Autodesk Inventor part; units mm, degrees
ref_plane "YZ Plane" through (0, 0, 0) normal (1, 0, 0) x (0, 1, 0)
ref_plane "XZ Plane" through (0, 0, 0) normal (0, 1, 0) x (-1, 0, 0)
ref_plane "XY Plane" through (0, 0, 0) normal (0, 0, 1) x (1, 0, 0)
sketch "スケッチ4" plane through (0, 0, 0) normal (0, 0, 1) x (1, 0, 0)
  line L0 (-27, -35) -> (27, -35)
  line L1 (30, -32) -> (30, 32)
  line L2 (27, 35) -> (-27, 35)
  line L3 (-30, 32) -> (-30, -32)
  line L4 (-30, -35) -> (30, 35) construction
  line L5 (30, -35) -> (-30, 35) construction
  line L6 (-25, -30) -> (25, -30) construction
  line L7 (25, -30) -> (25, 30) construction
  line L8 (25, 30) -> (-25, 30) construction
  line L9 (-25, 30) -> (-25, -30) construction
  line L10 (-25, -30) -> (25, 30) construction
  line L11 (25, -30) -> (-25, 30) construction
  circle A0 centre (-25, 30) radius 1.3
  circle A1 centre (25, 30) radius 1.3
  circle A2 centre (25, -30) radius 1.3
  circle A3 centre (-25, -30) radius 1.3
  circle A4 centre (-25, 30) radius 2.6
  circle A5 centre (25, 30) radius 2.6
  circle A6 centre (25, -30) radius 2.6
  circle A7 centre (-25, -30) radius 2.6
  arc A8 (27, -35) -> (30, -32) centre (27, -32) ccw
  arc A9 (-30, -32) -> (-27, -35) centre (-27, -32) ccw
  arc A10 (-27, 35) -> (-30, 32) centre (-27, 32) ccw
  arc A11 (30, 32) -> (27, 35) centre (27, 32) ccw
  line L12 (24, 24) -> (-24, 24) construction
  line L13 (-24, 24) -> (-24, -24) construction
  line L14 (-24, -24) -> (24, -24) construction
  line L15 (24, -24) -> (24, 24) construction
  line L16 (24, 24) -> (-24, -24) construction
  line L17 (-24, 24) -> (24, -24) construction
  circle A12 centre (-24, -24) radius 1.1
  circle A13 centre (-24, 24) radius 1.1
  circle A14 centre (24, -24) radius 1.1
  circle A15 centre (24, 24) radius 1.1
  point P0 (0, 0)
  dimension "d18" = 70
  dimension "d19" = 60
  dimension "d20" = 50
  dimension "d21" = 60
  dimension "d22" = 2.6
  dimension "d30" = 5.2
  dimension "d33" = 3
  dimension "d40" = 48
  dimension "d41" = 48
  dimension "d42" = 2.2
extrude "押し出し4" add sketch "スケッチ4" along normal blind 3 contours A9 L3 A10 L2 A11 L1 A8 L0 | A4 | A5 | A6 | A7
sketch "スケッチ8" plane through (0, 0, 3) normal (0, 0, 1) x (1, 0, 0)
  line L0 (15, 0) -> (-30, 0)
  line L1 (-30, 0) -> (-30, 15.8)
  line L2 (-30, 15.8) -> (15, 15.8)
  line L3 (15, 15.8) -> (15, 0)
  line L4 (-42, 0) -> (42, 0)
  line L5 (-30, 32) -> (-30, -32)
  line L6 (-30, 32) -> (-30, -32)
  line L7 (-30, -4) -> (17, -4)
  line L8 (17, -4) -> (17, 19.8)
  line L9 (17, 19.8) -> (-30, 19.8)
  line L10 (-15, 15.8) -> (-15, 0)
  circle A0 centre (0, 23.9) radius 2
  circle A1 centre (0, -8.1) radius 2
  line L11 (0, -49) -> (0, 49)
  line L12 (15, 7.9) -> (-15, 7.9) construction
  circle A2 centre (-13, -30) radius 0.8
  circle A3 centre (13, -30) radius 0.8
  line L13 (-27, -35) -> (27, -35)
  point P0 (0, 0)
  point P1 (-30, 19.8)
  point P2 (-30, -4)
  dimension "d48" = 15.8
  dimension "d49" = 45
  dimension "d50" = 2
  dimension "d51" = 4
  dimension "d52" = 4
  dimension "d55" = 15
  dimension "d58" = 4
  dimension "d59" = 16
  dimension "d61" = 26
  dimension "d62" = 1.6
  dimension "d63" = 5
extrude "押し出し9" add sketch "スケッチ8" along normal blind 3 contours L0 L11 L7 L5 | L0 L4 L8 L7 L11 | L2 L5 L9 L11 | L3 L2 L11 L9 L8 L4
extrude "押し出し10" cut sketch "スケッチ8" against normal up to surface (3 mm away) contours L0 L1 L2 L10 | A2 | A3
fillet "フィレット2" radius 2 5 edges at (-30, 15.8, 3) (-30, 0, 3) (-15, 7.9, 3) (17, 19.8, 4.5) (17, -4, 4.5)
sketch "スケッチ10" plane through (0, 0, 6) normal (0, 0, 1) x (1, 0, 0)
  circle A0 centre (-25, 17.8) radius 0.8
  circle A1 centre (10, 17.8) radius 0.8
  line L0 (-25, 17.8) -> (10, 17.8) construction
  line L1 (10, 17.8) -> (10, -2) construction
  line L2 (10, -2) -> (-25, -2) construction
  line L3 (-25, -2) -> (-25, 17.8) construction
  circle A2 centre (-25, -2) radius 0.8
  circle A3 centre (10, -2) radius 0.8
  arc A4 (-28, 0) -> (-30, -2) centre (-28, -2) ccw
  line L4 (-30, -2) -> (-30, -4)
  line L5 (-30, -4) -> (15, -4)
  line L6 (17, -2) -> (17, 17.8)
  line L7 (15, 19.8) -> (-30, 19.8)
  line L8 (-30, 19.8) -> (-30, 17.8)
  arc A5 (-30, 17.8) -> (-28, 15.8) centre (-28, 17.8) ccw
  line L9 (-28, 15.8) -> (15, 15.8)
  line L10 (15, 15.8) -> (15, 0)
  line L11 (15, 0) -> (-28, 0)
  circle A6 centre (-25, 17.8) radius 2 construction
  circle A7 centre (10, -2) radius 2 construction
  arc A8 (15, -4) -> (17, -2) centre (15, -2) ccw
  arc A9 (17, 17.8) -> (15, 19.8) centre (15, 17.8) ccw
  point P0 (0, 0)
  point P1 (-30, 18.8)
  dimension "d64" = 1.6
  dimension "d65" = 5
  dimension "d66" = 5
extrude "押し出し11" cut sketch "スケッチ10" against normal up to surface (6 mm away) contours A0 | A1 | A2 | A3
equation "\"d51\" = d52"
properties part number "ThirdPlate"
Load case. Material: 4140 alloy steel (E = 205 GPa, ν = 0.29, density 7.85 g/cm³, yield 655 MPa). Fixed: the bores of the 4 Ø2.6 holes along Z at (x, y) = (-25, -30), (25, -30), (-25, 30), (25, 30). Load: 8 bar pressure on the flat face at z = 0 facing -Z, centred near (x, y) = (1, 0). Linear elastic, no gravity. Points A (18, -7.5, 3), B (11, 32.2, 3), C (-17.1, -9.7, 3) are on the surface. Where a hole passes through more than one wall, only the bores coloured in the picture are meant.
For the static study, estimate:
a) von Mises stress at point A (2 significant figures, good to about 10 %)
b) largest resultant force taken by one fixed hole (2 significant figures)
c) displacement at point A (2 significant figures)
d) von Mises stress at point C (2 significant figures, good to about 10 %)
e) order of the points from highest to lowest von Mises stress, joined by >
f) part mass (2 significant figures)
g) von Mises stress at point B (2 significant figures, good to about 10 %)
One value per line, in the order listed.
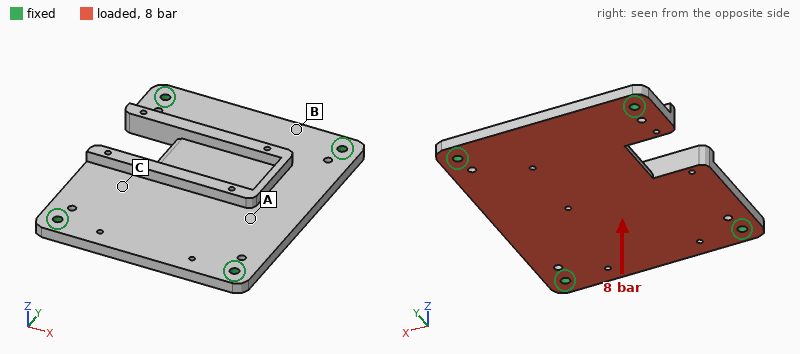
100 MPa
860 N
0.089 mm
74 MPa
A > C > B
100 g
32 MPa
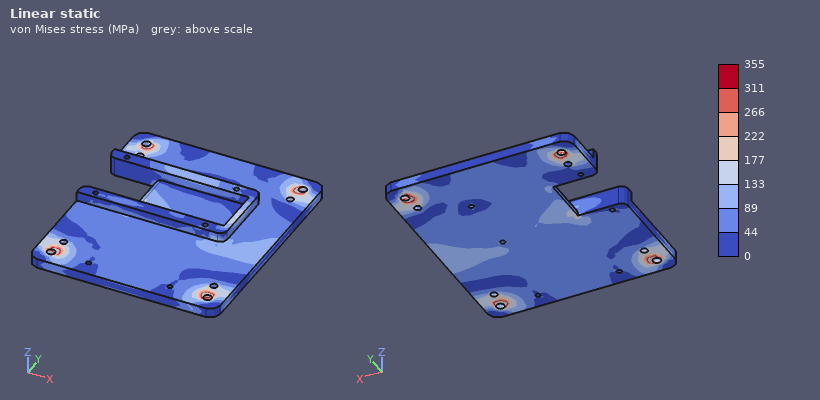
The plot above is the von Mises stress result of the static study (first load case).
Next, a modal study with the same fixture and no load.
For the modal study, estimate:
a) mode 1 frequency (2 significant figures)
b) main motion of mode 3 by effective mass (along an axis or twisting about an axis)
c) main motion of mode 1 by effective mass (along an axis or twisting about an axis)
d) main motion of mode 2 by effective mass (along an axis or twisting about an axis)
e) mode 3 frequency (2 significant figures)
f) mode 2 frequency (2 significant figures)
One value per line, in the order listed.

3000 Hz
twisting about X
along Z
twisting about Y
6300 Hz
4900 Hz
